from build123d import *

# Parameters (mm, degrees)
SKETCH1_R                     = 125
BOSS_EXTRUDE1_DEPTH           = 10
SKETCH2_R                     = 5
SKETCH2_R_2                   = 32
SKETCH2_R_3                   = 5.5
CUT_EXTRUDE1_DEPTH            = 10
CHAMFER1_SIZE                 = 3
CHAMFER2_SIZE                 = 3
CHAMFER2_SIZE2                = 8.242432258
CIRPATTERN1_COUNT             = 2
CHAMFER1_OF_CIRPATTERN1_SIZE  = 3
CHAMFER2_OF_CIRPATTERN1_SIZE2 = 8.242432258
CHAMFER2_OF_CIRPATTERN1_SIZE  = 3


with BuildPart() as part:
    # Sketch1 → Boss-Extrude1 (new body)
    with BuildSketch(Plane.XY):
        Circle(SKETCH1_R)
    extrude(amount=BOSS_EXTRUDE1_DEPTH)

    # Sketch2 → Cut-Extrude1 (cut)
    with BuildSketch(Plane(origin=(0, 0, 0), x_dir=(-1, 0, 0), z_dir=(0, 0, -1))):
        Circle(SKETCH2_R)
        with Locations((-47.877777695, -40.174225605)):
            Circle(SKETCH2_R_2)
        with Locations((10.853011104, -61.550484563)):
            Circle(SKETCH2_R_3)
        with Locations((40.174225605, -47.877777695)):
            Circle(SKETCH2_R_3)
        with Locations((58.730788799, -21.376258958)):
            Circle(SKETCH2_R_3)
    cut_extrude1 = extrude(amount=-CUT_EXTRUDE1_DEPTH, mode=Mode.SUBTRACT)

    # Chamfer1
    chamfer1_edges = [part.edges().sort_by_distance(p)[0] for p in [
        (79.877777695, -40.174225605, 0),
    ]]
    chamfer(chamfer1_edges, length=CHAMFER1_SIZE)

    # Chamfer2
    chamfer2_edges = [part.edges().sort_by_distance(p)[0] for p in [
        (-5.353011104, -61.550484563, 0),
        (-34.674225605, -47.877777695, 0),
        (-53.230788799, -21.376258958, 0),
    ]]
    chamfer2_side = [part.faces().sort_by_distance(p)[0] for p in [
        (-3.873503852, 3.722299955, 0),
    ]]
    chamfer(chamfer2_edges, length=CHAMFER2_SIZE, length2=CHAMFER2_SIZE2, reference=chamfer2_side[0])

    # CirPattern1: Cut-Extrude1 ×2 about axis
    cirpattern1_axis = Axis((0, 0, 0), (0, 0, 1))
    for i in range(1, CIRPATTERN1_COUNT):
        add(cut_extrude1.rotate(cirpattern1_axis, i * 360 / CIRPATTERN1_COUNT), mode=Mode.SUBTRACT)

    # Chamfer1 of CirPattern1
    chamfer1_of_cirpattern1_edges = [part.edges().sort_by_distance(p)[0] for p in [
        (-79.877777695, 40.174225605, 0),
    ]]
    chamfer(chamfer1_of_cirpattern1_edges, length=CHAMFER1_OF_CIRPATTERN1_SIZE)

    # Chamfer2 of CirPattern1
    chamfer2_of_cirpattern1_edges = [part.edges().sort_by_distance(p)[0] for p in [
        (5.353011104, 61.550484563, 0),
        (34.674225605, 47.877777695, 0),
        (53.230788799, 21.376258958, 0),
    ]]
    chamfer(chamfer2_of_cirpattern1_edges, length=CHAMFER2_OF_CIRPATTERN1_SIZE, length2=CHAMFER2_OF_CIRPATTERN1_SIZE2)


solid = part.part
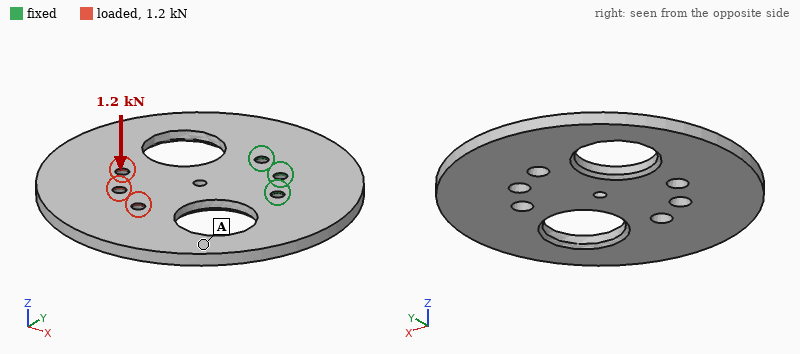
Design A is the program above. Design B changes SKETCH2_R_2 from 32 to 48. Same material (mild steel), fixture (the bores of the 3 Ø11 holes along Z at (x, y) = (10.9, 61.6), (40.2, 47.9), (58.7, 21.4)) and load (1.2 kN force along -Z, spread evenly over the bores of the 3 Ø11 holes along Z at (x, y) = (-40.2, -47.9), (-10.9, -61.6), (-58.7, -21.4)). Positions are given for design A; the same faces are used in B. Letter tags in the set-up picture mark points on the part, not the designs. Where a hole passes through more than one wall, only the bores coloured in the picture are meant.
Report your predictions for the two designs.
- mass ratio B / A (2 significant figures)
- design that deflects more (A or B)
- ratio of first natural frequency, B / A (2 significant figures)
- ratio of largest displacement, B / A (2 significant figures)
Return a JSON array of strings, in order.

["0.80", "B", "0.79", "1.7"]
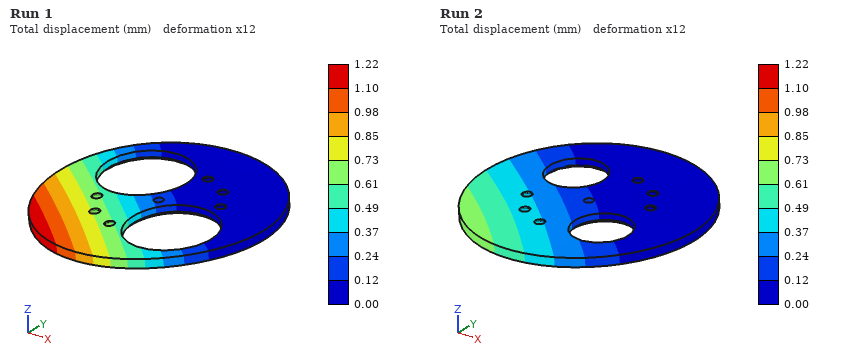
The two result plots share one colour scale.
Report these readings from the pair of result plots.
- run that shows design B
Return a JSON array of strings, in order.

["Run 1"]
